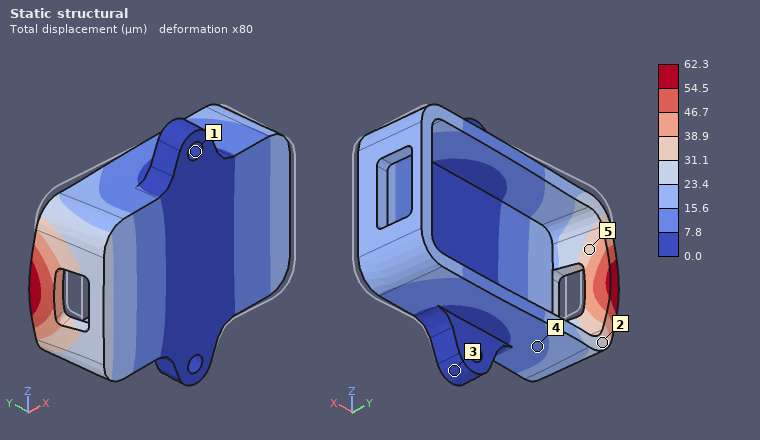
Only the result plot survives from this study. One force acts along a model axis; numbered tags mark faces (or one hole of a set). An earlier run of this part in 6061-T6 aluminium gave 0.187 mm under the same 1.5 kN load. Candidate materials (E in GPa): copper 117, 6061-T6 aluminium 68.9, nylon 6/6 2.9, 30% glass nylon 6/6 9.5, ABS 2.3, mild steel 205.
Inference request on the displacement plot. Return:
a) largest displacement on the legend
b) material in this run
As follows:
62.3 µm
mild steel
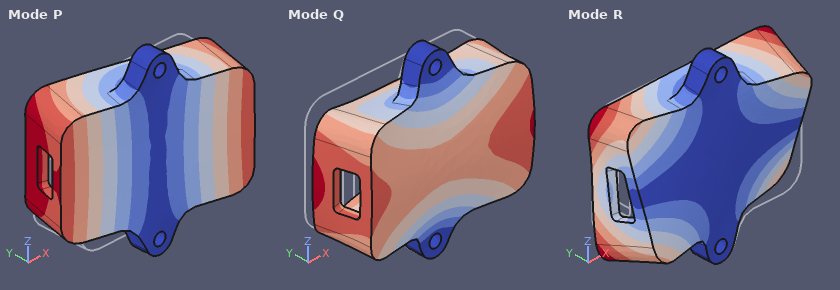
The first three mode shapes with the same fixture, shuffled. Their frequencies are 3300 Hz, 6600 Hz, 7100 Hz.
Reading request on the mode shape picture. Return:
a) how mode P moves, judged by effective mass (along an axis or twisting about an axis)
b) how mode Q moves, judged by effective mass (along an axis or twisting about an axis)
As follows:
twisting about Z
along Y
